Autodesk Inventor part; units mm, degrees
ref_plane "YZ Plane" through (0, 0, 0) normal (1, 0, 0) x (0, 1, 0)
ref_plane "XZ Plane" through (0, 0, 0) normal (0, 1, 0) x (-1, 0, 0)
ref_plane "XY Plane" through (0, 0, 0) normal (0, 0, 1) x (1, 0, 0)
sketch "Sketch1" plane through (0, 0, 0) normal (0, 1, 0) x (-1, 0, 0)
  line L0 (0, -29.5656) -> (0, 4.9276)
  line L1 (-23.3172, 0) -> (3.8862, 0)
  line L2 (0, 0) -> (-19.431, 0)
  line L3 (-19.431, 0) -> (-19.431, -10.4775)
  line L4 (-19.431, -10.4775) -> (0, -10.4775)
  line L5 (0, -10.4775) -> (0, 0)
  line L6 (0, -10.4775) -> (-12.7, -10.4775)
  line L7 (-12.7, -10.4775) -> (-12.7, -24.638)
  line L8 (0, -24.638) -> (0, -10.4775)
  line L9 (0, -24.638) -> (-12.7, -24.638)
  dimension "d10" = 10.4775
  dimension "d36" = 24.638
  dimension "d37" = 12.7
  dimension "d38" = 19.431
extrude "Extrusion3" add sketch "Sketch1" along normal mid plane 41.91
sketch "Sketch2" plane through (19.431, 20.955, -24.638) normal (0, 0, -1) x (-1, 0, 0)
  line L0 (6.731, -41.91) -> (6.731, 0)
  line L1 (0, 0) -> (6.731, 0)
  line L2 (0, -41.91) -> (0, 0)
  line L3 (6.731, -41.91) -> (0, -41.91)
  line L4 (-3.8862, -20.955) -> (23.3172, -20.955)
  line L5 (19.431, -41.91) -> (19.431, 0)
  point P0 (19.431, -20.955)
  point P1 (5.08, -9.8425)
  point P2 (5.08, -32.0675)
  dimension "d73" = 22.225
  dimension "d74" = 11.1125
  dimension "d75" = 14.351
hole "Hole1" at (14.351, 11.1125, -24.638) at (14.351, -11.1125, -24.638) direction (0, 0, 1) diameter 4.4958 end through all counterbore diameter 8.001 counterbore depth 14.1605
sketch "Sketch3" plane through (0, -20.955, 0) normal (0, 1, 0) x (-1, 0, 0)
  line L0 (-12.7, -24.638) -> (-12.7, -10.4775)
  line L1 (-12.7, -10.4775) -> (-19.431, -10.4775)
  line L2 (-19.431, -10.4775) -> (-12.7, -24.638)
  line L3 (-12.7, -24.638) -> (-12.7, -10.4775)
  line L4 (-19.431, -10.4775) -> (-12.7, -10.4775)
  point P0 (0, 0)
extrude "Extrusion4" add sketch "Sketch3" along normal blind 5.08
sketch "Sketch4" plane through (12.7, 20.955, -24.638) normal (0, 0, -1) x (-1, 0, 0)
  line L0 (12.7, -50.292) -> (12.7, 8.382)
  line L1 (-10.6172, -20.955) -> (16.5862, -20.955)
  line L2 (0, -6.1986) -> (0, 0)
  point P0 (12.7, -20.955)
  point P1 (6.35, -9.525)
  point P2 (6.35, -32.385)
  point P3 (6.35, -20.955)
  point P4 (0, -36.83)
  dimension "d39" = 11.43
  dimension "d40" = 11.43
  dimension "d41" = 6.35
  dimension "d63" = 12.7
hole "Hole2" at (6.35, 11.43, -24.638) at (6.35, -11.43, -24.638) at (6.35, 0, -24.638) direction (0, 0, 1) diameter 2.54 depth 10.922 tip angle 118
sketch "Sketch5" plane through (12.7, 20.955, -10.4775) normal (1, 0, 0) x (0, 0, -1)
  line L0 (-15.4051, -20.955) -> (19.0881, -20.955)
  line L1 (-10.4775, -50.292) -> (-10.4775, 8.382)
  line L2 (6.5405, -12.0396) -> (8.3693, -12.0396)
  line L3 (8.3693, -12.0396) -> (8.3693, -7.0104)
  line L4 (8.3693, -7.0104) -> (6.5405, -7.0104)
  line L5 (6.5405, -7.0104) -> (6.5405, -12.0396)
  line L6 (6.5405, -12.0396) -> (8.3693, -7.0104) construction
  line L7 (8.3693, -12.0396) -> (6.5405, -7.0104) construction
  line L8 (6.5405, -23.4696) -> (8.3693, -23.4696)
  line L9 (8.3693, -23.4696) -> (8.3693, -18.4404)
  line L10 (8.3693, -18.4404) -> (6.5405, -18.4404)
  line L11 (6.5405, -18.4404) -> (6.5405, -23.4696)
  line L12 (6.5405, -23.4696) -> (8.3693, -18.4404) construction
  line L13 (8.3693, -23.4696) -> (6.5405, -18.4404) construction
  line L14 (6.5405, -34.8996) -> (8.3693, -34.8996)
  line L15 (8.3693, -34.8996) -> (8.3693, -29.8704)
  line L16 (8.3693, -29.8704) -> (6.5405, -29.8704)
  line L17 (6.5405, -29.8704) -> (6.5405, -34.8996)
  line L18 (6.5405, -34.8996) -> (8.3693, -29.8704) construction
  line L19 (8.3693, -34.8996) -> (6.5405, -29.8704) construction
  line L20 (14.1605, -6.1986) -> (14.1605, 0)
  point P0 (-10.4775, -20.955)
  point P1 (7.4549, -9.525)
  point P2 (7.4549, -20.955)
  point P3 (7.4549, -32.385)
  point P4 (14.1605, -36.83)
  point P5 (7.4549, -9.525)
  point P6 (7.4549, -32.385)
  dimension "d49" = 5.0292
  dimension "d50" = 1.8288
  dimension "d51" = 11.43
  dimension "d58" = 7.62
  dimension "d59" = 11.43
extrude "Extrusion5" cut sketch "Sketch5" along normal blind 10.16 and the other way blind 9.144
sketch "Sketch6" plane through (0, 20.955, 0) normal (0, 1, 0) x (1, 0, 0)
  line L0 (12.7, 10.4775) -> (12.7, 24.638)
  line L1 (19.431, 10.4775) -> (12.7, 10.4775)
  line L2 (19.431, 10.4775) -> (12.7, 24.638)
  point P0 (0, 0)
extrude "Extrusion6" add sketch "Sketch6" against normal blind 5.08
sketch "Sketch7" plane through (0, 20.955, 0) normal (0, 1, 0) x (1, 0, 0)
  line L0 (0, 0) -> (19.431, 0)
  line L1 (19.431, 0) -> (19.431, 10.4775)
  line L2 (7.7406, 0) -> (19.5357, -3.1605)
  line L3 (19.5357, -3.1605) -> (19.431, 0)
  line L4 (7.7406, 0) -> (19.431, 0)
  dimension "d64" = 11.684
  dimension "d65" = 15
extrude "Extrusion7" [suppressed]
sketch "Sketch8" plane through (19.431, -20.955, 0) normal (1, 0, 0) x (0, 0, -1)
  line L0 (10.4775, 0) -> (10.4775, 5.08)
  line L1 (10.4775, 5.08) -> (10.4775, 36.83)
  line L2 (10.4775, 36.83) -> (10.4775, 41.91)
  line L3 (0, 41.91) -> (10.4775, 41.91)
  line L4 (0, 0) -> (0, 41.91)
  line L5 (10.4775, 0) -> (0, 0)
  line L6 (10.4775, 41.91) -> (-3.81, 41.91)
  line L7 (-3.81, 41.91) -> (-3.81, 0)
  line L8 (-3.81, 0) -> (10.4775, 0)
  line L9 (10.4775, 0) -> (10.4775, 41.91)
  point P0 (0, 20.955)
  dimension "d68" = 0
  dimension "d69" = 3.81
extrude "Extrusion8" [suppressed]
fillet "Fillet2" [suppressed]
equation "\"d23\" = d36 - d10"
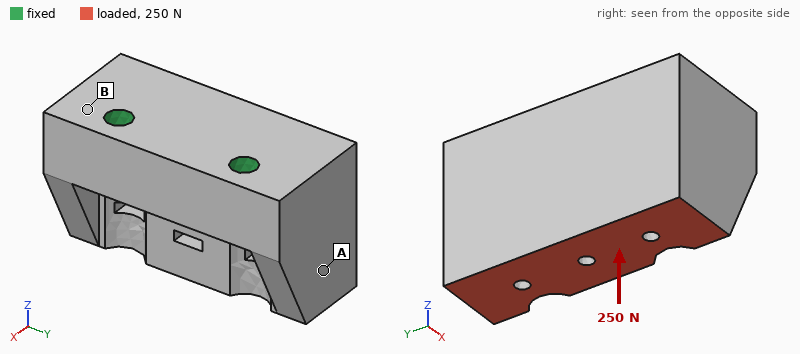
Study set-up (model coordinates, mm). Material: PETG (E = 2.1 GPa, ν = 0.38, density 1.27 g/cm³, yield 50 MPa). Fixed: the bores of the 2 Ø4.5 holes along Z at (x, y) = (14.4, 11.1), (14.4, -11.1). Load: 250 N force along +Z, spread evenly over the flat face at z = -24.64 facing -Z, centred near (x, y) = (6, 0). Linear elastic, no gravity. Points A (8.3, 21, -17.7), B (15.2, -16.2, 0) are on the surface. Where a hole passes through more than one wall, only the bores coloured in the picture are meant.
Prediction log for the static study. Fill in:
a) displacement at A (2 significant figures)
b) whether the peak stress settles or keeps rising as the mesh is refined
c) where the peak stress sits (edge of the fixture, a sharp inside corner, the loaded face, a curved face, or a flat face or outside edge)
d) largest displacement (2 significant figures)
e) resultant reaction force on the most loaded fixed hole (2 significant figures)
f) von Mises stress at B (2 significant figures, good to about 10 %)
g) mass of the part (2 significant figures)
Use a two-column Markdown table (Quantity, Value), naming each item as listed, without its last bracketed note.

| Quantity | Value |
|---|---|
| displacement at A | 23 µm |
| whether the peak stress settles or keeps rising as the mesh is refined | keeps rising |
| where the peak stress sits | edge of the fixture |
| largest displacement | 42 µm |
| resultant reaction force on the most loaded fixed hole | 130 N |
| von Mises stress at B | 1.1 MPa |
| mass of the part | 20 g |
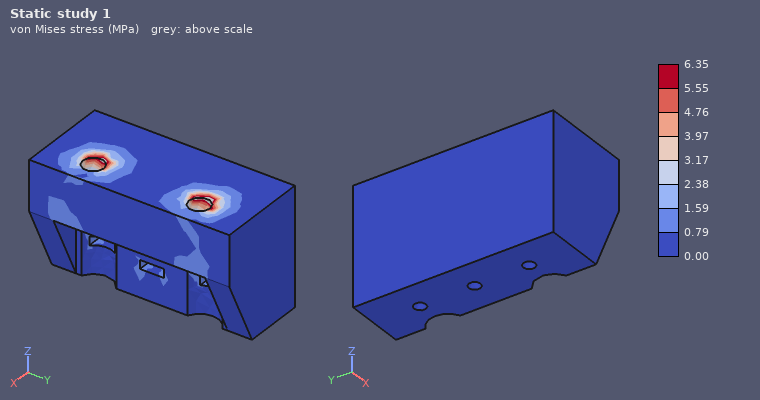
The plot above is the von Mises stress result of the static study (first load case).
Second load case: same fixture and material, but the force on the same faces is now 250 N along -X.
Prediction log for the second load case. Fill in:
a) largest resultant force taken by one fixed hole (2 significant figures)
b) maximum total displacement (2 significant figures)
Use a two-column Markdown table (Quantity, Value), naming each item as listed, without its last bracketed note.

| Quantity | Value |
|---|---|
| largest resultant force taken by one fixed hole | 130 N |
| maximum total displacement | 0.14 mm |
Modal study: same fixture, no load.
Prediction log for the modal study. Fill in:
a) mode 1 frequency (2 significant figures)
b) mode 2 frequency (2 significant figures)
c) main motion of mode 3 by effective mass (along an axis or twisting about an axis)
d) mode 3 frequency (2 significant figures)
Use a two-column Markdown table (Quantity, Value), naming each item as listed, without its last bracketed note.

| Quantity | Value |
|---|---|
| mode 1 frequency | 3200 Hz |
| mode 2 frequency | 4600 Hz |
| main motion of mode 3 by effective mass | along Y |
| mode 3 frequency | 5700 Hz |
